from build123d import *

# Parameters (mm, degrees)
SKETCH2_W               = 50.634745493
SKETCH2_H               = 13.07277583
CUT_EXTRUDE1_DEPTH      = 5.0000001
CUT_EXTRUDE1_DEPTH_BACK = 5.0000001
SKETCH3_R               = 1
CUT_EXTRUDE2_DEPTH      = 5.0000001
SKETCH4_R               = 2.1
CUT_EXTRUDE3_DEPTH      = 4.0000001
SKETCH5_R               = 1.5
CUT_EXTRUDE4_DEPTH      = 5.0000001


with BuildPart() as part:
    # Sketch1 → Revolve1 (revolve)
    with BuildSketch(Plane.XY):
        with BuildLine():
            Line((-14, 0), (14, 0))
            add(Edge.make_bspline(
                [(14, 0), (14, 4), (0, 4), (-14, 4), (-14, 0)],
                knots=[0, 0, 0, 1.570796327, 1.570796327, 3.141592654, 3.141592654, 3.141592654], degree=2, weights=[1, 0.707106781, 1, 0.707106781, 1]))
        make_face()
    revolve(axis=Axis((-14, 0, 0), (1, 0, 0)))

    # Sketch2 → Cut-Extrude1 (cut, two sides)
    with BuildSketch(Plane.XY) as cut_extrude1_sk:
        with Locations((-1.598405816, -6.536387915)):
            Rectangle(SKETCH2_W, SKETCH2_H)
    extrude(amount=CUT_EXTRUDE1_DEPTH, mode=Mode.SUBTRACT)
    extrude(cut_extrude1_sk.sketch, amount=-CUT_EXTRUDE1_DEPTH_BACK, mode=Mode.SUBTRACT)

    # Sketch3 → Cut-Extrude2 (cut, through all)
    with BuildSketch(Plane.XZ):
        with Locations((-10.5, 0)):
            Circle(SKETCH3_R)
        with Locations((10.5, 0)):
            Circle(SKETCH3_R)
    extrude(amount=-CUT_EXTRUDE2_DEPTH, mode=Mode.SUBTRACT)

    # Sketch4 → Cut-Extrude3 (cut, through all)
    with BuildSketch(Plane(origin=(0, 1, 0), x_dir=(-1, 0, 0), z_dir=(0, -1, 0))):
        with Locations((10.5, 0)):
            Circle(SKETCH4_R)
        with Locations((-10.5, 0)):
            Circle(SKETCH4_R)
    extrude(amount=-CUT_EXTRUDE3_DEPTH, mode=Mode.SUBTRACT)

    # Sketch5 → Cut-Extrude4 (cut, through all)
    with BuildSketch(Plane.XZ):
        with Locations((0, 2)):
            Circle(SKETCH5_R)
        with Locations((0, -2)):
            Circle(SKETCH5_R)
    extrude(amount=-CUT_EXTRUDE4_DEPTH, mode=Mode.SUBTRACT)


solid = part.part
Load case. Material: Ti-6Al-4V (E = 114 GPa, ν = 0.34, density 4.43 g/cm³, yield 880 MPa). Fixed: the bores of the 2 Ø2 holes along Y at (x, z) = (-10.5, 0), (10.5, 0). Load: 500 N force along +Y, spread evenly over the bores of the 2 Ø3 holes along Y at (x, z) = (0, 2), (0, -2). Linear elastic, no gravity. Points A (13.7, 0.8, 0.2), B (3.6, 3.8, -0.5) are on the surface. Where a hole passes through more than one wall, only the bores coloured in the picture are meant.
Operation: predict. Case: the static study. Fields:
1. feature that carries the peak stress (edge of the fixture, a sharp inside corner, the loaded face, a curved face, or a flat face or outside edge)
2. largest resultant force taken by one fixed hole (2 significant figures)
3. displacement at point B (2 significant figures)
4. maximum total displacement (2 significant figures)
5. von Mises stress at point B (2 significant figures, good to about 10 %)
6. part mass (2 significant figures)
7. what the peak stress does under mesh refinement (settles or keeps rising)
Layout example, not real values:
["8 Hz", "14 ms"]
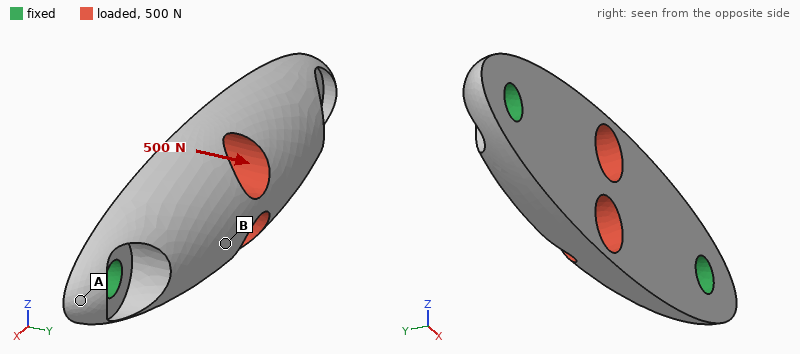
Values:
["edge of the fixture", "530 N", "25 µm", "36 µm", "120 MPa", "1.7 g", "keeps rising"]
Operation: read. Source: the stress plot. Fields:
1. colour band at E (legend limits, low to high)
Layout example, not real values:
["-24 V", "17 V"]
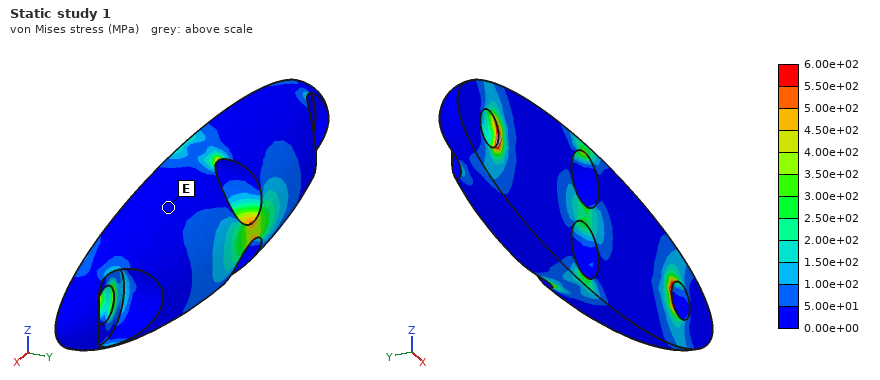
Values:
["0.00e+00 to 5.00e+01 MPa"]
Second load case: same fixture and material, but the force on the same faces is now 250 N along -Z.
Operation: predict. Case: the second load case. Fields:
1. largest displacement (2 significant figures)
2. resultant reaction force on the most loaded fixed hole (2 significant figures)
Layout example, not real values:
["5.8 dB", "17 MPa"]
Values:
["13 µm", "130 N"]
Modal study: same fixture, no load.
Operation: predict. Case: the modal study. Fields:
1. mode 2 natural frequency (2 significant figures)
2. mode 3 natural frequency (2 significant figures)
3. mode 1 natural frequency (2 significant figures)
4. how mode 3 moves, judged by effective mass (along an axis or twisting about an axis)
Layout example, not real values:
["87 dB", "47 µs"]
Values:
["23 kHz", "34 kHz", "23 kHz", "along Z"]
